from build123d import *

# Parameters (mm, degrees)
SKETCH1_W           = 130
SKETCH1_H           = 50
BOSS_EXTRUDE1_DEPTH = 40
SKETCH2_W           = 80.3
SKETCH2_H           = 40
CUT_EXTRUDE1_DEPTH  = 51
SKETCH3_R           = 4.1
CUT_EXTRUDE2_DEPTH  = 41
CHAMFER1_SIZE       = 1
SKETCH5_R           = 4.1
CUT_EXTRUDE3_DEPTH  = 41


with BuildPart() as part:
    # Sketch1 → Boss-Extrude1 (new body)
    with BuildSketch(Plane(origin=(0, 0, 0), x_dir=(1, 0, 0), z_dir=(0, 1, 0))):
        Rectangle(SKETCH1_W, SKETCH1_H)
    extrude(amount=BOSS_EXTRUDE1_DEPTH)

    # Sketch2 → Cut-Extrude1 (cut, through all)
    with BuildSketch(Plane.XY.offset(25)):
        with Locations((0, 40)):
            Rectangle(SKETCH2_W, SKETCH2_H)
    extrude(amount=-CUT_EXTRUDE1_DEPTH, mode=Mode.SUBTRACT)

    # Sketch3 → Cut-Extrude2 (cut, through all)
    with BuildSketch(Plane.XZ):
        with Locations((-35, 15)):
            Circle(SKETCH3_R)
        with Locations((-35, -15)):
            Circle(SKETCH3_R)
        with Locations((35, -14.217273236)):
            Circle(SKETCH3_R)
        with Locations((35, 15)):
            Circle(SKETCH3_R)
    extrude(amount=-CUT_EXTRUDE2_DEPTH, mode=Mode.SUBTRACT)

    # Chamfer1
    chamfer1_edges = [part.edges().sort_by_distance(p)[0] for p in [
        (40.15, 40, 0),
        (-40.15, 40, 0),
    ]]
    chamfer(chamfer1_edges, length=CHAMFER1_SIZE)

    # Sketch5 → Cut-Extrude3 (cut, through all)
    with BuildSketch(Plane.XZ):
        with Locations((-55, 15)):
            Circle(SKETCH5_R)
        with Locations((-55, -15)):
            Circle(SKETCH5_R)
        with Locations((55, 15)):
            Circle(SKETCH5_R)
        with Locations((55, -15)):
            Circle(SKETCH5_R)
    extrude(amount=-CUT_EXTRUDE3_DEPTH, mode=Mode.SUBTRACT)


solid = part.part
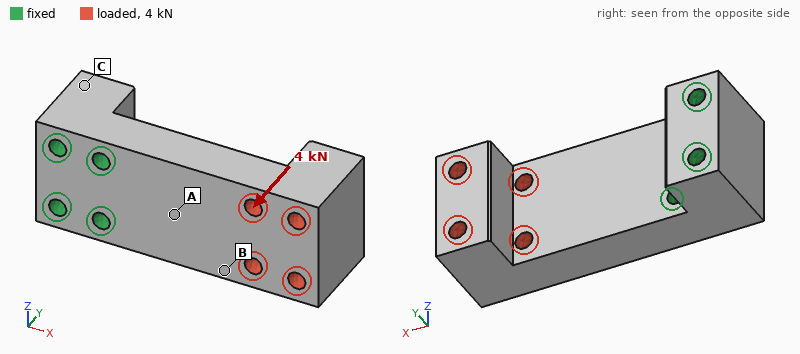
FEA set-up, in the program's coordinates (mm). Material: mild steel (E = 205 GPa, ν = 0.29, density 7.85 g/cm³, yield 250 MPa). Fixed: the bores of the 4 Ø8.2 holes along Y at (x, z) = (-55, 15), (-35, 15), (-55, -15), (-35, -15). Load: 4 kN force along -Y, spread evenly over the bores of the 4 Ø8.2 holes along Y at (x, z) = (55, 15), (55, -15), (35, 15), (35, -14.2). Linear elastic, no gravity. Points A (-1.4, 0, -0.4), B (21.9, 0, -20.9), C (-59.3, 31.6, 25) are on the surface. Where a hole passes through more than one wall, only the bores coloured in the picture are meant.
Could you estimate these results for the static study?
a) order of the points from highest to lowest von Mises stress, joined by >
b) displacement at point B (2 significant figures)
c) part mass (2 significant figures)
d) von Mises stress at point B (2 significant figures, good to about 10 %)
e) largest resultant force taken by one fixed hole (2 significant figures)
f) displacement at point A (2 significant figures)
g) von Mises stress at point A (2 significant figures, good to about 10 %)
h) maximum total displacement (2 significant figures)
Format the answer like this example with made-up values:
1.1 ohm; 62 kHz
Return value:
A > B > C; 0.064 mm; 1.3 kg; 33 MPa; 2.9 kN; 0.029 mm; 58 MPa; 0.16 mm
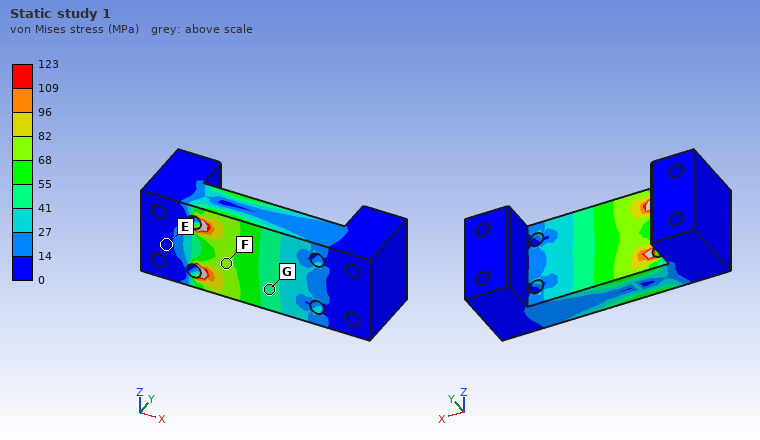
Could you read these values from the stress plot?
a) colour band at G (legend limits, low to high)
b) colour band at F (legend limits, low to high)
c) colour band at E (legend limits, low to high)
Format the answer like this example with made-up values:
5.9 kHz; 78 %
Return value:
41 to 55 MPa; 68 to 82 MPa; 0 to 14 MPa
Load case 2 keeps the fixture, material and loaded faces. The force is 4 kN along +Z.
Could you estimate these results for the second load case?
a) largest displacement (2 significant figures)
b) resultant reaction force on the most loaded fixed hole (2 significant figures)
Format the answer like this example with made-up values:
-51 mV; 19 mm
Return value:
37 µm; 8.9 kN
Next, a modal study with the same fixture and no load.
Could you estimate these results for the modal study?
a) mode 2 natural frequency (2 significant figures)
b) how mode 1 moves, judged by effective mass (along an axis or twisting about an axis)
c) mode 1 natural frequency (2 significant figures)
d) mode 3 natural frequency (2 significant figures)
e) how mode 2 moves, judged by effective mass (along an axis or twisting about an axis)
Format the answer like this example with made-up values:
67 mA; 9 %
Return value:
2700 Hz; along Y; 1300 Hz; 4300 Hz; along Z
